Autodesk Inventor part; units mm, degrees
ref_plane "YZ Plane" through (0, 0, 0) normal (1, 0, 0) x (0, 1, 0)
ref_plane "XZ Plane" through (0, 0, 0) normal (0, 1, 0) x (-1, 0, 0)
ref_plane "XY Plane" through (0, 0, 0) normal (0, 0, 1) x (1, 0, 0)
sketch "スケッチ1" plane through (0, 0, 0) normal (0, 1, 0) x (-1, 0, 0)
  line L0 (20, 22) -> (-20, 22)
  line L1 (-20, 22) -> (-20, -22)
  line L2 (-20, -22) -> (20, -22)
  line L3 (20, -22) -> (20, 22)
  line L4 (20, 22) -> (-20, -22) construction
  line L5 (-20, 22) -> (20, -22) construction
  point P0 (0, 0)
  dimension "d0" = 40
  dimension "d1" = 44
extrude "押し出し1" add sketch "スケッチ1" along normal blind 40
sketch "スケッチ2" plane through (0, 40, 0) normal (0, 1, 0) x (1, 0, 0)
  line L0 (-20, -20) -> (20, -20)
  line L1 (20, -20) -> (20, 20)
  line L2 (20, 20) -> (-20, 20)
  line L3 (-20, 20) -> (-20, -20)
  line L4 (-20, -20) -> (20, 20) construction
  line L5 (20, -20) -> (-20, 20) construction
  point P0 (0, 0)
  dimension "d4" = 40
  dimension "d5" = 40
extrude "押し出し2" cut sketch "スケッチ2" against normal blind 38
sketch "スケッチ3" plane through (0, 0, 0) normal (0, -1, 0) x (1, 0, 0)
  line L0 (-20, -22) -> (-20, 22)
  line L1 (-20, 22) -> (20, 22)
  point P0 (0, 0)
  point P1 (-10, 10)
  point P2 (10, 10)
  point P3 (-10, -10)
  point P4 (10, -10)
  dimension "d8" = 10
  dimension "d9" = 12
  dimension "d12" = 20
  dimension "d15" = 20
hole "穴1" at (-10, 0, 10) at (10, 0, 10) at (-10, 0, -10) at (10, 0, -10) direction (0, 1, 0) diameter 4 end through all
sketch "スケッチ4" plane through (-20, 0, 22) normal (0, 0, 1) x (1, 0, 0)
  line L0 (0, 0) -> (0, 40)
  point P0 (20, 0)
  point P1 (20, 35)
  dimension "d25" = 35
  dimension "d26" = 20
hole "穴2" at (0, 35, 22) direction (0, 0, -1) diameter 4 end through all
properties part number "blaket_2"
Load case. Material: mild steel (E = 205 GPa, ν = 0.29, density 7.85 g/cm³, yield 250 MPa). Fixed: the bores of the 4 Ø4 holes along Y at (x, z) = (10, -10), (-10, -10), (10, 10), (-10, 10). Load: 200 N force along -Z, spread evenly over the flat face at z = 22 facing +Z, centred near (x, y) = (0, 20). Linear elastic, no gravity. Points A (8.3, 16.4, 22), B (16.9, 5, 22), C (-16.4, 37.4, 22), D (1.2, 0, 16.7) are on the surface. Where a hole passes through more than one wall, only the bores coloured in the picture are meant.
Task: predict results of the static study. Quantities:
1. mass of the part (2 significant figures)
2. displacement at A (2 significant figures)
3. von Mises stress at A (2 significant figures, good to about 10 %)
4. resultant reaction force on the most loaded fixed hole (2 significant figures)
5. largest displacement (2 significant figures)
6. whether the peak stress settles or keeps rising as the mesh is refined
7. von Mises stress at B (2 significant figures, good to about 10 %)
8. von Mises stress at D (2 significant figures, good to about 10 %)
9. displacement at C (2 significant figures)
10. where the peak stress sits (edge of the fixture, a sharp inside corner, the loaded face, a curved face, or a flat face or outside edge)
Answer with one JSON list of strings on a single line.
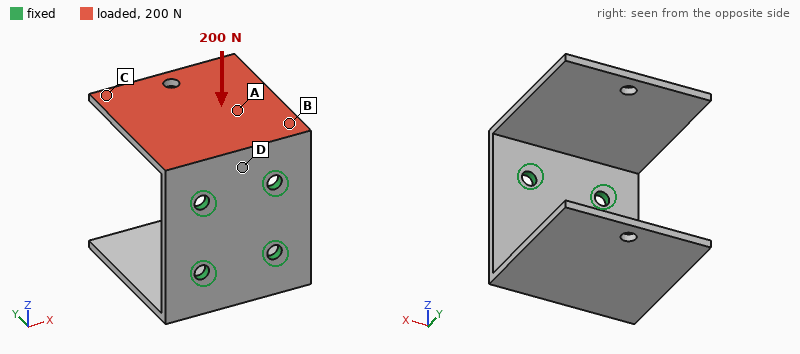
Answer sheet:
["74 g", "0.17 mm", "47 MPa", "90 N", "0.50 mm", "keeps rising", "100 MPa", "120 MPa", "0.46 mm", "edge of the fixture"]
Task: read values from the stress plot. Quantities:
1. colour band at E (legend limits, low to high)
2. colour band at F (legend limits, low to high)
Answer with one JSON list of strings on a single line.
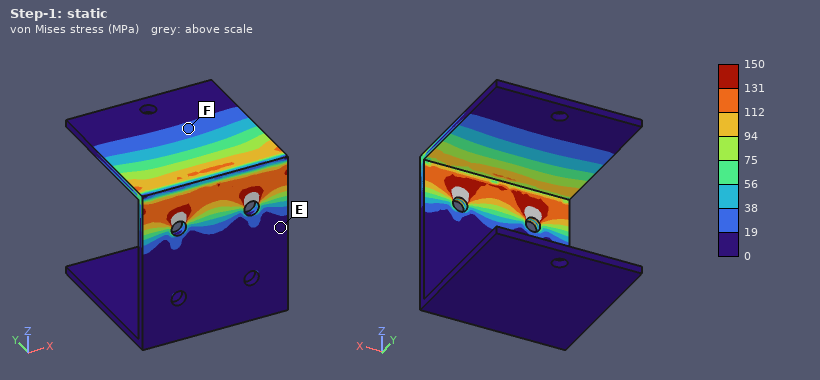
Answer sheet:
["0 to 19 MPa", "19 to 38 MPa"]
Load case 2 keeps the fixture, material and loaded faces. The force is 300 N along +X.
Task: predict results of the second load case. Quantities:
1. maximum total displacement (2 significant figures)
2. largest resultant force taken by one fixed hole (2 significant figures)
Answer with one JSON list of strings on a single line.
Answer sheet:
["78 µm", "310 N"]
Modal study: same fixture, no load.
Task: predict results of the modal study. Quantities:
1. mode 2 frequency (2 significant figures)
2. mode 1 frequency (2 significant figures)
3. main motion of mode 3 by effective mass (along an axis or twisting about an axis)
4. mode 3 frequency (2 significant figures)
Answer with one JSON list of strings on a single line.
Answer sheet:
["790 Hz", "780 Hz", "along X", "2000 Hz"]
